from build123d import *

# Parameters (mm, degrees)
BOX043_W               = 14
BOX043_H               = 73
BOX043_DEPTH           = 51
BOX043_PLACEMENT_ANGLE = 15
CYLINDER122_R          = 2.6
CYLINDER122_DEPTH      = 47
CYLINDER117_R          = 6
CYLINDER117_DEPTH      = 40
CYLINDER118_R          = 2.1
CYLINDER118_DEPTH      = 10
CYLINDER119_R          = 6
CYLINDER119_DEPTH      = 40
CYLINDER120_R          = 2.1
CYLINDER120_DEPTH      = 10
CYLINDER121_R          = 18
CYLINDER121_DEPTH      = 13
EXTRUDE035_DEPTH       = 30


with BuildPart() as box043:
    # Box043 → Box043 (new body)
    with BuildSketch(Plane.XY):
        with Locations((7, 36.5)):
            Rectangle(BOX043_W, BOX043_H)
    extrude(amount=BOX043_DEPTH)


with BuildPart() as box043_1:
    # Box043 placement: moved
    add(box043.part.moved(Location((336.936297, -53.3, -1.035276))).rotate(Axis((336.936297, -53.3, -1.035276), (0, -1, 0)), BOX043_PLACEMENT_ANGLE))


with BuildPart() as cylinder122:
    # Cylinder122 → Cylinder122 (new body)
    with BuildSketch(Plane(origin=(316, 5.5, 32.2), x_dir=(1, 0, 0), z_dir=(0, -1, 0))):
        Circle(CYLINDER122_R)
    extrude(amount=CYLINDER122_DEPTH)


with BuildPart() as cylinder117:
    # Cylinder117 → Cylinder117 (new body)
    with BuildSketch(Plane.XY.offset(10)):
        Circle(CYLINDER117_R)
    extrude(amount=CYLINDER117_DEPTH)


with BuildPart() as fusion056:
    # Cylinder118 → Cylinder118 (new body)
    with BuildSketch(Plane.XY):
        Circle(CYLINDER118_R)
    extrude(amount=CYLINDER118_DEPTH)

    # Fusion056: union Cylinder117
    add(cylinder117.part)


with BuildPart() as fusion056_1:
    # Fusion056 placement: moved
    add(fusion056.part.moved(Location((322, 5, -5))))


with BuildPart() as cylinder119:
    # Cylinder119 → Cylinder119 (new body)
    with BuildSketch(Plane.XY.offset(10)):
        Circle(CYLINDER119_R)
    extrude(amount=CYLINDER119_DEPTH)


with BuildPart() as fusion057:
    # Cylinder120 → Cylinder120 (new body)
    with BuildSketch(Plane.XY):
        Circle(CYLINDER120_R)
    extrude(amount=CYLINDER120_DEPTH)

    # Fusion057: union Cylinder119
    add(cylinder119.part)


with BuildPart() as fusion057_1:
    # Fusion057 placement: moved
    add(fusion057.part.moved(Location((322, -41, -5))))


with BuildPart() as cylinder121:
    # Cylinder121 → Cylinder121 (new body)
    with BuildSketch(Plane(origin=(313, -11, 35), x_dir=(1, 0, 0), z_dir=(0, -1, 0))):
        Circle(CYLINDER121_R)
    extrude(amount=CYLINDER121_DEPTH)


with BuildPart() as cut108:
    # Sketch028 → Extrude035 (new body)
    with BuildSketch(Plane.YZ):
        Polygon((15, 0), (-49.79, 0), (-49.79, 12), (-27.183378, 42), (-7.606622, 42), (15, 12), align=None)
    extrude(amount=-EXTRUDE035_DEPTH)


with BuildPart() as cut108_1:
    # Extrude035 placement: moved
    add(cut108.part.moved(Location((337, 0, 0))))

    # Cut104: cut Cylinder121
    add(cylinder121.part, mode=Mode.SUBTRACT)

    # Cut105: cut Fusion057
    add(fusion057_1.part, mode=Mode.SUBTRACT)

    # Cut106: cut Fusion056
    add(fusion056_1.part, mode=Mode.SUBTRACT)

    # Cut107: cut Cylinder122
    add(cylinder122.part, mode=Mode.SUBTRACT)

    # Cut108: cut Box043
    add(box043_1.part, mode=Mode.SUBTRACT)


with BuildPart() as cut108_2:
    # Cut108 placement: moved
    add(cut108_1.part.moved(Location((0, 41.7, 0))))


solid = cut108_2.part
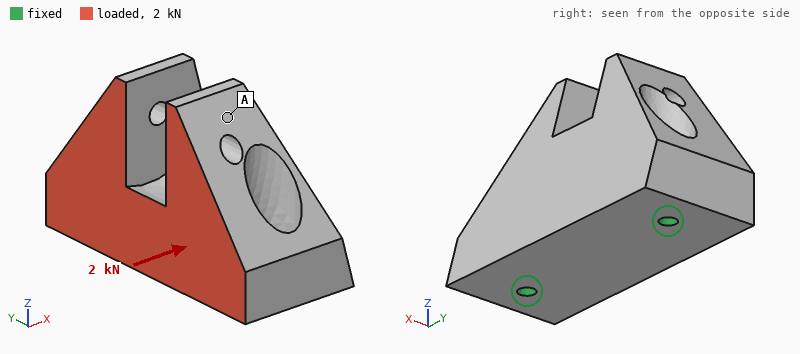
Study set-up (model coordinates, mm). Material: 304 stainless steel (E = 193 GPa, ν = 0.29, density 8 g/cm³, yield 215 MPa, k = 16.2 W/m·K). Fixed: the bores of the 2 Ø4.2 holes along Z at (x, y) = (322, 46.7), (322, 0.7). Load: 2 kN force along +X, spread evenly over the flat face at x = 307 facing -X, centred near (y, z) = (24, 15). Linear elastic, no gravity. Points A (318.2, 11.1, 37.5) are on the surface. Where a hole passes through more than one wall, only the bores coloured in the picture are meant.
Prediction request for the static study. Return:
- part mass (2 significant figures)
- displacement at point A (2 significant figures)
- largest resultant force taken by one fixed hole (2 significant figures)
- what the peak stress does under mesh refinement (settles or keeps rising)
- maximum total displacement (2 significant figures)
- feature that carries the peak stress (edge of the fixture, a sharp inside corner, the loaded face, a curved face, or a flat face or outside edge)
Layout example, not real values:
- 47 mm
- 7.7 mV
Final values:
- 320 g
- 28 µm
- 1.0 kN
- keeps rising
- 33 µm
- edge of the fixture
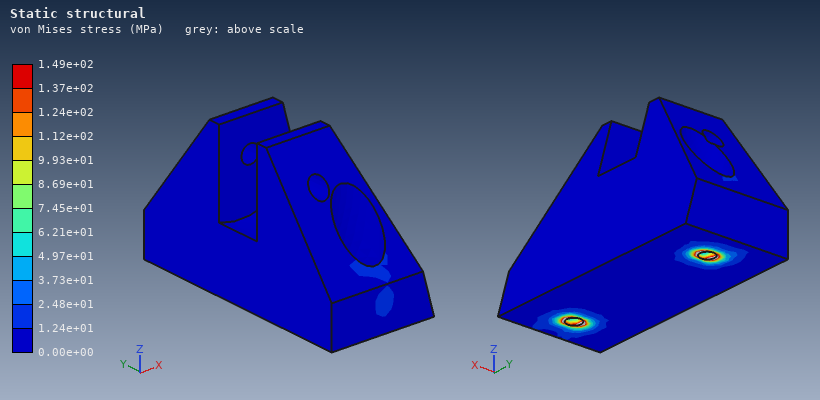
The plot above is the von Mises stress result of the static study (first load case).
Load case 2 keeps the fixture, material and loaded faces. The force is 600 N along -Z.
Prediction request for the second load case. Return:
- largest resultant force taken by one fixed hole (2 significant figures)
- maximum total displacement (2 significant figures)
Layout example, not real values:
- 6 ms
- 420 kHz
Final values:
- 320 N
- 12 µm
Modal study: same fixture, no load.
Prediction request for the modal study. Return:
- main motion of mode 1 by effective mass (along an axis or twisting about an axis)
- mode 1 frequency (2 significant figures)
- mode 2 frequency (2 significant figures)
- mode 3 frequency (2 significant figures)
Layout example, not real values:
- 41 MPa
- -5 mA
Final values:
- along X
- 3000 Hz
- 11 kHz
- 11 kHz
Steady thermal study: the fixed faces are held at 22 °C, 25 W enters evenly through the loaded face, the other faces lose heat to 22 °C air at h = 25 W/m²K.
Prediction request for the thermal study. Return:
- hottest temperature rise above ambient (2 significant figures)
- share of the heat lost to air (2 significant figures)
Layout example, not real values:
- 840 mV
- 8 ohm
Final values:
- 50 K
- 29 %
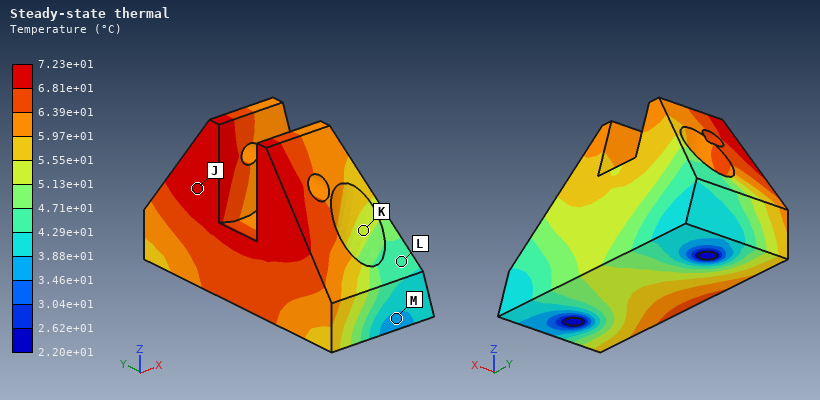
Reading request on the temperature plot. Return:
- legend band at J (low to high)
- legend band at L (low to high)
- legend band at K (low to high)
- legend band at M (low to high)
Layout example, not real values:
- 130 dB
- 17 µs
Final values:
- 6.81e+01 to 7.23e+01 °C
- 4.29e+01 to 4.71e+01 °C
- 5.13e+01 to 5.55e+01 °C
- 3.46e+01 to 3.88e+01 °C
